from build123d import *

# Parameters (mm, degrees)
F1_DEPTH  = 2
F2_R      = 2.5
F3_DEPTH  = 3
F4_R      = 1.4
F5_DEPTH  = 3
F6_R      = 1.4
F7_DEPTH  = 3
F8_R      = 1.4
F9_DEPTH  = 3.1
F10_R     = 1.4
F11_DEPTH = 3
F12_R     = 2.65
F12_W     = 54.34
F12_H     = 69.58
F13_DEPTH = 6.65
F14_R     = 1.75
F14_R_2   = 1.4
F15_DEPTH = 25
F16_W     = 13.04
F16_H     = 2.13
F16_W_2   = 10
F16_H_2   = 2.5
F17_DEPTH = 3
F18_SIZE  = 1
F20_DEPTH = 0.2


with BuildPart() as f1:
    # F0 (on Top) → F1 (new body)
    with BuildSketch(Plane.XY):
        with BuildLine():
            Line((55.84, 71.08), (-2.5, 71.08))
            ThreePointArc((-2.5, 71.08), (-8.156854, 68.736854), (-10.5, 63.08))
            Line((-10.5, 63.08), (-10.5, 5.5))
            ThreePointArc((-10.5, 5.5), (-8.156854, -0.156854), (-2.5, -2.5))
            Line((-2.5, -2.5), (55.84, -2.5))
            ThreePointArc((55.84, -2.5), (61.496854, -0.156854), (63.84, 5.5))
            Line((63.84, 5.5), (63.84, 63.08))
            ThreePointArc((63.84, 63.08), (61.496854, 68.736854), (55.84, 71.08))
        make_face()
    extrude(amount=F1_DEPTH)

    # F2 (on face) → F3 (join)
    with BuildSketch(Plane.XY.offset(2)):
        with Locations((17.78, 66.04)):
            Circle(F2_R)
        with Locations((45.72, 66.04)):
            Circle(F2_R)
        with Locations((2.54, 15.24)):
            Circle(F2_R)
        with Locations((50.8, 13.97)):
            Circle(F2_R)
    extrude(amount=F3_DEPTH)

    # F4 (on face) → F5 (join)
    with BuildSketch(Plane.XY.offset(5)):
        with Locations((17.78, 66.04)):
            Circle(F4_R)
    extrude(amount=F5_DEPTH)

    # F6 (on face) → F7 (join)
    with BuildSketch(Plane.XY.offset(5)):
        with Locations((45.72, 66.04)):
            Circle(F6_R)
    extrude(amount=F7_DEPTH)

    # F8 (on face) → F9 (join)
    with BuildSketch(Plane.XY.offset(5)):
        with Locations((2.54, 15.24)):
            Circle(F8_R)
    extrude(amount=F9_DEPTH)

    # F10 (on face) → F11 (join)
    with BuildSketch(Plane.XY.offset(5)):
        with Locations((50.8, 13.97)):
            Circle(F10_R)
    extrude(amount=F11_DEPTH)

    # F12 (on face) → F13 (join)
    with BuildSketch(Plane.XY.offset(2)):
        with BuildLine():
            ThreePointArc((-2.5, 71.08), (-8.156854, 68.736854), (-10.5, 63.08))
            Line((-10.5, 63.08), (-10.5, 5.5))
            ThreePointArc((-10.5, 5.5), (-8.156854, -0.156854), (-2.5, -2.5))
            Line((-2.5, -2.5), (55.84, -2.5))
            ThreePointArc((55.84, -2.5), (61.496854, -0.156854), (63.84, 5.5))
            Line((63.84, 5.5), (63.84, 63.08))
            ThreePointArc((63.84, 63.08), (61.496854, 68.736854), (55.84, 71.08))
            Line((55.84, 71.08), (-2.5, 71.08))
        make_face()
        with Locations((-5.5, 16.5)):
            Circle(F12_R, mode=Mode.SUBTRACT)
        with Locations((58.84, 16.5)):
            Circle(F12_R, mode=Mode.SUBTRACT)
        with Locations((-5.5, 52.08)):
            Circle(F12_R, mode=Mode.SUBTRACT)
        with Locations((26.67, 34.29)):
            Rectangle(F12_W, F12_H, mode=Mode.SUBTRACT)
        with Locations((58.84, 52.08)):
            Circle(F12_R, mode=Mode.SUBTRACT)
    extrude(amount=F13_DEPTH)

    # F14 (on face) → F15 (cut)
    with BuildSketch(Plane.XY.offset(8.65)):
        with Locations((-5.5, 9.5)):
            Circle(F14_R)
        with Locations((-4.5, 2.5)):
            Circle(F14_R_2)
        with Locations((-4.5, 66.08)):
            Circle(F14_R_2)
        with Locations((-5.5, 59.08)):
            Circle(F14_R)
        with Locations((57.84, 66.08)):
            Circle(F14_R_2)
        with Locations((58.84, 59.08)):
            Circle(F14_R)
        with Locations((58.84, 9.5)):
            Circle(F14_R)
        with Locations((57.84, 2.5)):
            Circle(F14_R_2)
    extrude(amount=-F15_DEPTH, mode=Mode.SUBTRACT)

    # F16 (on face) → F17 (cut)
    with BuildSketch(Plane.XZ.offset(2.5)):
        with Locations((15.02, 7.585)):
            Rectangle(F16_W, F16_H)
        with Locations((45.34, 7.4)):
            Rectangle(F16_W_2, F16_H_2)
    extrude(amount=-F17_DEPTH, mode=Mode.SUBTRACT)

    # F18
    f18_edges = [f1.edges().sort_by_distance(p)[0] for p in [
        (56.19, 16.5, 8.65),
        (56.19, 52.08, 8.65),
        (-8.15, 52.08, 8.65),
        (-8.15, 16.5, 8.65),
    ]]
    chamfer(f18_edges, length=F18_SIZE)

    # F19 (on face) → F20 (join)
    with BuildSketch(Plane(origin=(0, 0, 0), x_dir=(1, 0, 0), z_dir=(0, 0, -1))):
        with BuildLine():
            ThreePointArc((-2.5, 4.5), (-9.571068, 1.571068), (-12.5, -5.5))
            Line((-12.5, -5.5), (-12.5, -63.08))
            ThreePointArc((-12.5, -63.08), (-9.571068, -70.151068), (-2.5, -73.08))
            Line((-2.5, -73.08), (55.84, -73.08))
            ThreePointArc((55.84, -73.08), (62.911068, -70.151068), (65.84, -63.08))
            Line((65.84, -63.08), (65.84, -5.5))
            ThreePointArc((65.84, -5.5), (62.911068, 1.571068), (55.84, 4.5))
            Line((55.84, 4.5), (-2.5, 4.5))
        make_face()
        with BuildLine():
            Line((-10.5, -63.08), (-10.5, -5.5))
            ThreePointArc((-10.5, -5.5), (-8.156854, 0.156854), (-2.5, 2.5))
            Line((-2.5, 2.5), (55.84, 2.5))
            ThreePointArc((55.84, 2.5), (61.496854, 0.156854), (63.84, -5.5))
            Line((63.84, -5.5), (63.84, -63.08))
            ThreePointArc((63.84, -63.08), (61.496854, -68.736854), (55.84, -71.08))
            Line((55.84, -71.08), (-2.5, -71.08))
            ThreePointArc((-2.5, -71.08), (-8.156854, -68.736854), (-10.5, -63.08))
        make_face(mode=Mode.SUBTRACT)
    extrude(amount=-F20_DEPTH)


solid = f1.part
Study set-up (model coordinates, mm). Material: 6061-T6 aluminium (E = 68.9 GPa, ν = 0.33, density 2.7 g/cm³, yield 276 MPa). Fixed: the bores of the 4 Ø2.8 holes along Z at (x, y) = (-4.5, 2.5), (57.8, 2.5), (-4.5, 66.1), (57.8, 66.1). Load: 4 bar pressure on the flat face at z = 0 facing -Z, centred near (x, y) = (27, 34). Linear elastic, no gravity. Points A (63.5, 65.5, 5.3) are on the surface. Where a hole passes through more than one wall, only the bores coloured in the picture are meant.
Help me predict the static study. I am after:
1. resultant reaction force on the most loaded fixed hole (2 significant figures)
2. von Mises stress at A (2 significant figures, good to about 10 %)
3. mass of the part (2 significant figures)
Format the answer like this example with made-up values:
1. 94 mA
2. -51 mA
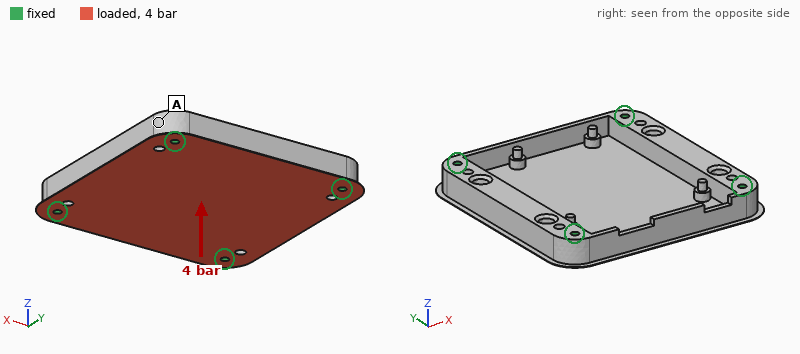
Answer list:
1. 690 N
2. 16 MPa
3. 56 g
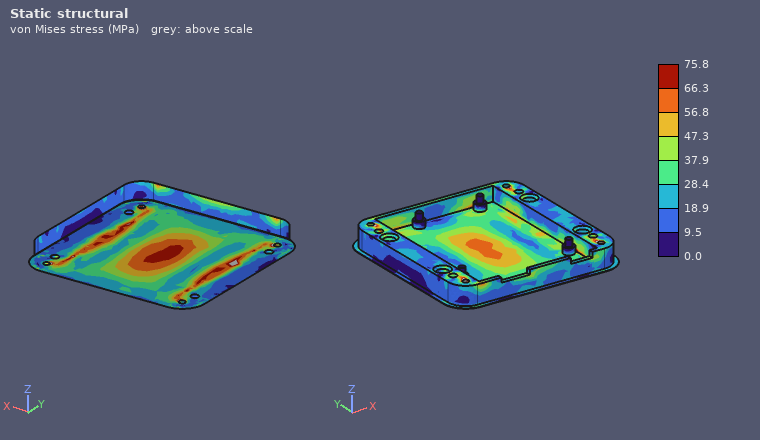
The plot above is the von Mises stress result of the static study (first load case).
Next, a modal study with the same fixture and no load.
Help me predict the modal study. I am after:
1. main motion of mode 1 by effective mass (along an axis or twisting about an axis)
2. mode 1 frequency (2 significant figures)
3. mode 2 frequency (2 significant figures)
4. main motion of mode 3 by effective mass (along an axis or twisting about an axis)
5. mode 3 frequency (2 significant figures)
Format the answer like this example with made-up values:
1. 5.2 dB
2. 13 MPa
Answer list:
1. along Z
2. 3700 Hz
3. 5900 Hz
4. twisting about Y
5. 7600 Hz
